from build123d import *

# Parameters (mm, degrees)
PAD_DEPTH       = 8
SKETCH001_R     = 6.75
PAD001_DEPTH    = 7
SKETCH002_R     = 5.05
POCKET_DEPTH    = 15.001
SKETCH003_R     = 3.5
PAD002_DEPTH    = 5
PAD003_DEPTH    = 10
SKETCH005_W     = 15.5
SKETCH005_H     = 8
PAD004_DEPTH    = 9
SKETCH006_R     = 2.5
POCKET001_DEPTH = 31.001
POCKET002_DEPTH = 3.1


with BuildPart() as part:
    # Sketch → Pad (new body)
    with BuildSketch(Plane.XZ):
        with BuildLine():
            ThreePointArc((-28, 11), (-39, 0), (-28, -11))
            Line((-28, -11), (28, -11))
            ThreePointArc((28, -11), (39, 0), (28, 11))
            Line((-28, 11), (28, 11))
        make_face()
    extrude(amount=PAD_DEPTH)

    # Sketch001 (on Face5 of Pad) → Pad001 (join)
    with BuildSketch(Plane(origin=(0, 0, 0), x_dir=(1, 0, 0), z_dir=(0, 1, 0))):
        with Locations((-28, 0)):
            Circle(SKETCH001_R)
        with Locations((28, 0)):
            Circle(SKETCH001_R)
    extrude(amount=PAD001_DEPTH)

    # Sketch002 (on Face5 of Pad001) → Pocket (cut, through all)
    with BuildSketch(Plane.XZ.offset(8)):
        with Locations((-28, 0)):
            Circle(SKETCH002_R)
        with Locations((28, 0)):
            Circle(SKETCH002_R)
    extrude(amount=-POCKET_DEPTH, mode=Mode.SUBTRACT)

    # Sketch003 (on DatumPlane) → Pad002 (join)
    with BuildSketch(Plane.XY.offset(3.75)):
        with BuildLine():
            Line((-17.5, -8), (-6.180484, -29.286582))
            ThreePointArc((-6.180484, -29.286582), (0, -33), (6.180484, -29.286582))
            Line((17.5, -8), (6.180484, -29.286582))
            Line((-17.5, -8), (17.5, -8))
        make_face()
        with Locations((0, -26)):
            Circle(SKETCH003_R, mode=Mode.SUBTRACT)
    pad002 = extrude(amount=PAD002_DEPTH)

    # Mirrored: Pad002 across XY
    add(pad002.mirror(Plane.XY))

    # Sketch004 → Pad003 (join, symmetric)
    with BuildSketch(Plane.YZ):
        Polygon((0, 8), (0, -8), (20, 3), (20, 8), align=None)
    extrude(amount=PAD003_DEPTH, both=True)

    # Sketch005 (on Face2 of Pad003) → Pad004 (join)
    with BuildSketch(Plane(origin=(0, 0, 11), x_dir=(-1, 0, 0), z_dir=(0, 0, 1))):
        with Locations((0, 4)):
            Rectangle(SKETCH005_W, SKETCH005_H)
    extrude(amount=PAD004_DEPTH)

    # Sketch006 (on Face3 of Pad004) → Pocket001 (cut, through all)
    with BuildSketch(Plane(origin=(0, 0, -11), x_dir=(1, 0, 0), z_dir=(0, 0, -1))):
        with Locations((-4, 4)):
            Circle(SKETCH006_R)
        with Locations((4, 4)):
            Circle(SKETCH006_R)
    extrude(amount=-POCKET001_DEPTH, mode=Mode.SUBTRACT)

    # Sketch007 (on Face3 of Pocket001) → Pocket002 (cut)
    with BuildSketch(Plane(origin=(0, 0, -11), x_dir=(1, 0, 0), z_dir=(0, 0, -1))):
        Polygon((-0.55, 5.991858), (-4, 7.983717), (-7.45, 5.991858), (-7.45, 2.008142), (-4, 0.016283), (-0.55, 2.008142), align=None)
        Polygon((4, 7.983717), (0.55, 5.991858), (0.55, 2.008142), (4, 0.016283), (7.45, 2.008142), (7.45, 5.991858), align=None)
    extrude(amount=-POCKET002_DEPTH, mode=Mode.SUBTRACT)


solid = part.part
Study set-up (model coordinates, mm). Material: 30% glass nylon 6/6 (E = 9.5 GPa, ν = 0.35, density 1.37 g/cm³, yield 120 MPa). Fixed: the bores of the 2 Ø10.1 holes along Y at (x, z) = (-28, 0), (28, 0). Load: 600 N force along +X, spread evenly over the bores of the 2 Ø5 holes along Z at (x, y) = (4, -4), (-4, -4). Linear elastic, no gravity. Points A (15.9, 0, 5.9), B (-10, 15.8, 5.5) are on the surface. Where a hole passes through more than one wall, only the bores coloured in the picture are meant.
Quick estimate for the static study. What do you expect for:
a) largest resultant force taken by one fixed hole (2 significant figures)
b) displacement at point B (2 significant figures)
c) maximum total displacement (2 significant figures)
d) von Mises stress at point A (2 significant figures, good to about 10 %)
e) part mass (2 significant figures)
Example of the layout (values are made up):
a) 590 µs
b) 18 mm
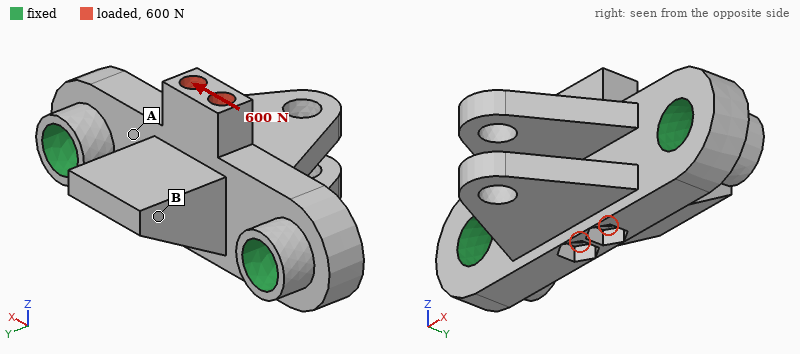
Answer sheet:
a) 310 N
b) 4.5 µm
c) 16 µm
d) 2.7 MPa
e) 29 g
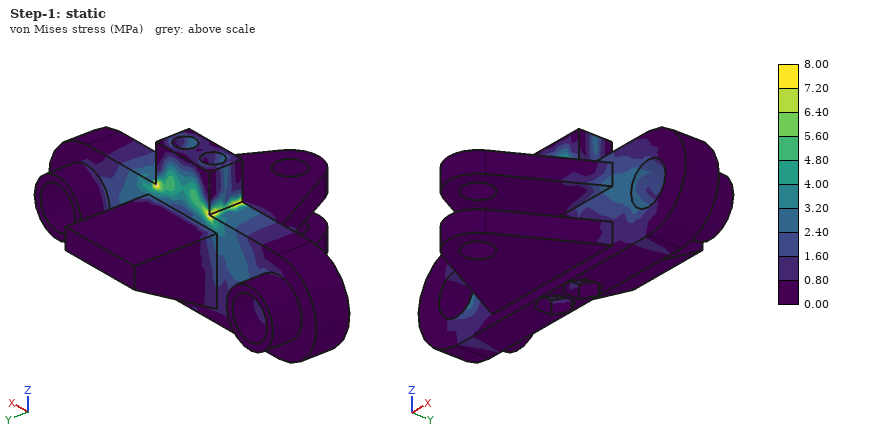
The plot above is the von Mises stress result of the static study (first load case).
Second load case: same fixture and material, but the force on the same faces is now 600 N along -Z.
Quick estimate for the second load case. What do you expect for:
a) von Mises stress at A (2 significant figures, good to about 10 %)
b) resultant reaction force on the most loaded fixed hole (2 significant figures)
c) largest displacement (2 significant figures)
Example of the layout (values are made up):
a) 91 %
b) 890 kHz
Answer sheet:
a) 3.3 MPa
b) 300 N
c) 24 µm
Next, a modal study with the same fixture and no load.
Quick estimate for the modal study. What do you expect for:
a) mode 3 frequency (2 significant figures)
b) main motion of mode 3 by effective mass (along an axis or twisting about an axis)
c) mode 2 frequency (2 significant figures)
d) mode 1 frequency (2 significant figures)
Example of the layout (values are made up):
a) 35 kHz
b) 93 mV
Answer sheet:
a) 5400 Hz
b) along Z
c) 4300 Hz
d) 3400 Hz
